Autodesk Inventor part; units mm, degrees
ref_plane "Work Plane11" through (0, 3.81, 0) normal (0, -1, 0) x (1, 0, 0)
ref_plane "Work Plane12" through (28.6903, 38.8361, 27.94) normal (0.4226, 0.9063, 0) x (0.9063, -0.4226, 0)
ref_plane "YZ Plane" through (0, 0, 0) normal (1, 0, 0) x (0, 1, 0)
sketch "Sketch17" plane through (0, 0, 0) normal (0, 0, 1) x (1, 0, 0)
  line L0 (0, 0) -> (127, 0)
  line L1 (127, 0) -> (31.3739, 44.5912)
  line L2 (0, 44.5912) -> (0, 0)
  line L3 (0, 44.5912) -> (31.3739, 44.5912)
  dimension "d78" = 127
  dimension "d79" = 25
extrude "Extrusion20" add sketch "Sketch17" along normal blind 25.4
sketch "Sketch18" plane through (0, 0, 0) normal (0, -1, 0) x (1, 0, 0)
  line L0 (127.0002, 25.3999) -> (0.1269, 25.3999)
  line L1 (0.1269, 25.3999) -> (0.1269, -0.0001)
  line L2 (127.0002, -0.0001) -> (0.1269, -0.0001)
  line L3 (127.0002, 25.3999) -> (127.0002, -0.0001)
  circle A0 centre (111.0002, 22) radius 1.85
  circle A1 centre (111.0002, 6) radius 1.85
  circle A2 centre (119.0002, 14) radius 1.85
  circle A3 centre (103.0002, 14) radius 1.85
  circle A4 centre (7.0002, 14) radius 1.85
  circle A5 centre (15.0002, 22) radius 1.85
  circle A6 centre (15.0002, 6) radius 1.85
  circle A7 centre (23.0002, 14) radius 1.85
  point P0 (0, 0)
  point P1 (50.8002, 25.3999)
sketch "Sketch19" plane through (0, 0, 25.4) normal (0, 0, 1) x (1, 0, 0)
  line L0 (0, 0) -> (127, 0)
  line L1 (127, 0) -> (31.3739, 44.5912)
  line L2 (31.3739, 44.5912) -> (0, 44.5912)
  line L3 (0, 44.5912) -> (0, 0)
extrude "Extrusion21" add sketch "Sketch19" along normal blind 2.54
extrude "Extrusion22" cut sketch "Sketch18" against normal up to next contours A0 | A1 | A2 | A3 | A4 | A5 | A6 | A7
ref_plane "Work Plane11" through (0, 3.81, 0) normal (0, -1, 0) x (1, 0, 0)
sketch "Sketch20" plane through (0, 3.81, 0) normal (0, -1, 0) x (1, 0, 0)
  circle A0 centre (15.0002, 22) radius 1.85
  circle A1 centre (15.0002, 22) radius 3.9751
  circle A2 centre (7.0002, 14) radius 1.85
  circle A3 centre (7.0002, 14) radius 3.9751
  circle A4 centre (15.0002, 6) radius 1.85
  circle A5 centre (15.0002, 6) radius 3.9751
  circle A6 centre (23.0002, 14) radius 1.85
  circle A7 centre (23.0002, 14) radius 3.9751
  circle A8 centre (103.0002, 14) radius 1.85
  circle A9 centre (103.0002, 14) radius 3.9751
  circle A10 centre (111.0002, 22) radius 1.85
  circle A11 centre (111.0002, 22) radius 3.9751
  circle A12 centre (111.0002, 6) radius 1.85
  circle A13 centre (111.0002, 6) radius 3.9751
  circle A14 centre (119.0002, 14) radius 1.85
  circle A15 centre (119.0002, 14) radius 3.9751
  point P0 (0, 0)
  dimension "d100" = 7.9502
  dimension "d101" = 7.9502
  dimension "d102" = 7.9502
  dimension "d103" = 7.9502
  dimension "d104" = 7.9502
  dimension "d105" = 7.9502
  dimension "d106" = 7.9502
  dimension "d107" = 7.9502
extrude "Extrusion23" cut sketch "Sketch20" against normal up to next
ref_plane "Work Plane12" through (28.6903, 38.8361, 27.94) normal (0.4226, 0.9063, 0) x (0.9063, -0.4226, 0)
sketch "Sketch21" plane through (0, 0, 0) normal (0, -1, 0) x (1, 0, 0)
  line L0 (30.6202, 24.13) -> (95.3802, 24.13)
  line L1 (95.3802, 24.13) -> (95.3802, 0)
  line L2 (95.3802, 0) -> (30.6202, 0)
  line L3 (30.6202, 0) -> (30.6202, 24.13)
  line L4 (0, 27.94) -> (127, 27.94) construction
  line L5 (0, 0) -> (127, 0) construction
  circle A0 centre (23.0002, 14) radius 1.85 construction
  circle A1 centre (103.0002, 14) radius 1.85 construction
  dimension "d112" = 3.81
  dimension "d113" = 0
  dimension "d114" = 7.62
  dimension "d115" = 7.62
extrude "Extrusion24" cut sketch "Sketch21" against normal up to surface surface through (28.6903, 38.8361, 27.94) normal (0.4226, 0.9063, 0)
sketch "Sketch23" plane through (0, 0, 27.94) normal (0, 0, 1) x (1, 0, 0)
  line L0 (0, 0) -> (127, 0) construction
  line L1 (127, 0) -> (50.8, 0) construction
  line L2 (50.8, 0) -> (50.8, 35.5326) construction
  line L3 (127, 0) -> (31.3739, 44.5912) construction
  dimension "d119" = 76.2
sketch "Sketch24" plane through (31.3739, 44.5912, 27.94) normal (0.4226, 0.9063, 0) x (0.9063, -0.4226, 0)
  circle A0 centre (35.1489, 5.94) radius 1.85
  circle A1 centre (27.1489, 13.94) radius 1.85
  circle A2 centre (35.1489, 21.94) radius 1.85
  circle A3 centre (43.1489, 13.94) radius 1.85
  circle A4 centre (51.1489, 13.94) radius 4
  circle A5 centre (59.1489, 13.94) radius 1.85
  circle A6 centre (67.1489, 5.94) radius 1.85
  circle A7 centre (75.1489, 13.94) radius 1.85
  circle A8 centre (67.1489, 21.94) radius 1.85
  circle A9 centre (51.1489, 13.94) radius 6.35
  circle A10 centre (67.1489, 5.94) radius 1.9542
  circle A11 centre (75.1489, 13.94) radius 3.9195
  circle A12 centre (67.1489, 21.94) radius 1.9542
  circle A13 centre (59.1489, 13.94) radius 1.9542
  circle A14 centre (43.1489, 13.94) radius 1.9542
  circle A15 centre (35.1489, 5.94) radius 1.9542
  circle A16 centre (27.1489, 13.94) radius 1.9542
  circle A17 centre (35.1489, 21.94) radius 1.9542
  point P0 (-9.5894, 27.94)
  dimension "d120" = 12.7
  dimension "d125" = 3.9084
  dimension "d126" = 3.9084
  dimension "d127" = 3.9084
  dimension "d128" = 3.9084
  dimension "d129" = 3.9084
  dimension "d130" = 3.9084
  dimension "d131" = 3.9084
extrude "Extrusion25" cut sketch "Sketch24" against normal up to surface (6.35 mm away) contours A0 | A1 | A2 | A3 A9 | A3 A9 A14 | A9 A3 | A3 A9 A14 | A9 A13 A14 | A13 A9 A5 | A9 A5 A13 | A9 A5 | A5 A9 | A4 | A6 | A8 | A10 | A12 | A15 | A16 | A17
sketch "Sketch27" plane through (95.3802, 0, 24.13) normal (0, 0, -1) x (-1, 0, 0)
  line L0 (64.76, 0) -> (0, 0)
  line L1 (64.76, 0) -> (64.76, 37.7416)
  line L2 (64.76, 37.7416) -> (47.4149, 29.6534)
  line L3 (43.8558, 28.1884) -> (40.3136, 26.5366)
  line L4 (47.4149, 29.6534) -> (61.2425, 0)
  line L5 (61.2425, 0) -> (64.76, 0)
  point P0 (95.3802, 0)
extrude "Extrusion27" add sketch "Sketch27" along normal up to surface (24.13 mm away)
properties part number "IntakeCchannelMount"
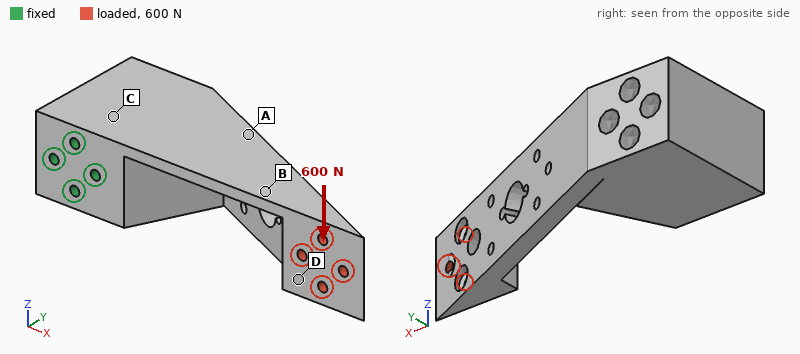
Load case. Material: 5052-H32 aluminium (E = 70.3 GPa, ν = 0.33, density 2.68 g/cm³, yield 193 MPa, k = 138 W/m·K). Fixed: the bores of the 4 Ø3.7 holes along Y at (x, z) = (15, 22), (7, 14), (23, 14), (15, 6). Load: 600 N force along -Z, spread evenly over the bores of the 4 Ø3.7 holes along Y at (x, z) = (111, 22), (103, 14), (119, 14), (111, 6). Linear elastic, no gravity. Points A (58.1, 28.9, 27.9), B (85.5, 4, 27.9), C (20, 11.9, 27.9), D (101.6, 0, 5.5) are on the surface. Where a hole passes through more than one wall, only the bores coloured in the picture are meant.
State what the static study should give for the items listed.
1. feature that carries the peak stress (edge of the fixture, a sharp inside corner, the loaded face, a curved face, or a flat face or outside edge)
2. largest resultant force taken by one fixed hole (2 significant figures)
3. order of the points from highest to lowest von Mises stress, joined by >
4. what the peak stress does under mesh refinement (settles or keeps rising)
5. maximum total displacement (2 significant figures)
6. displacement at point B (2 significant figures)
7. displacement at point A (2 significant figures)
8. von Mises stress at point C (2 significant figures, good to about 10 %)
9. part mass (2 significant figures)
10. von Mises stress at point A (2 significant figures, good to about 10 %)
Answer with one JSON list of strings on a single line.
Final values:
["edge of the fixture", "1.8 kN", "A > C > B > D", "keeps rising", "0.32 mm", "0.17 mm", "0.062 mm", "18 MPa", "170 g", "35 MPa"]
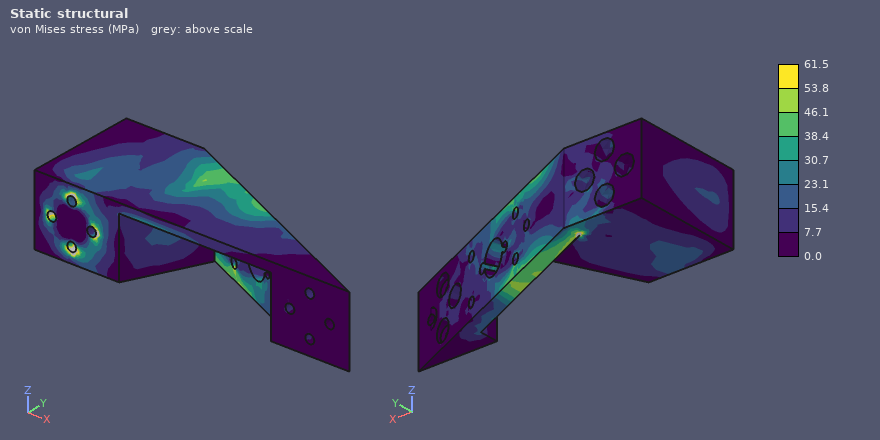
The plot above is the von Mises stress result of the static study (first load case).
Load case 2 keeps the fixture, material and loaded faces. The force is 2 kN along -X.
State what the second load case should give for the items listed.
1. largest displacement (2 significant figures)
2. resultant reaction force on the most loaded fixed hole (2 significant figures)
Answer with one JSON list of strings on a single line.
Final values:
["0.69 mm", "680 N"]
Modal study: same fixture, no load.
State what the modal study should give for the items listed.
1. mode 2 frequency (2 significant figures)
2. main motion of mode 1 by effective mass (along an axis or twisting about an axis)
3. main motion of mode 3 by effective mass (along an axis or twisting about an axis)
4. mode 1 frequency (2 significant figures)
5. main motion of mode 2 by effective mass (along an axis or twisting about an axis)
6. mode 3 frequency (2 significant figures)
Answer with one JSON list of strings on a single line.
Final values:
["1800 Hz", "along Y", "along X", "1400 Hz", "along Z", "2800 Hz"]
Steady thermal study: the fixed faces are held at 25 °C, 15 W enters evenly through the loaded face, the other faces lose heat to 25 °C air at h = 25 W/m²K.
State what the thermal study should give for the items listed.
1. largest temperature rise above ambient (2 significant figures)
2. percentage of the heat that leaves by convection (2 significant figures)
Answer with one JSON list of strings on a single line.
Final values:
["39 K", "36 %"]
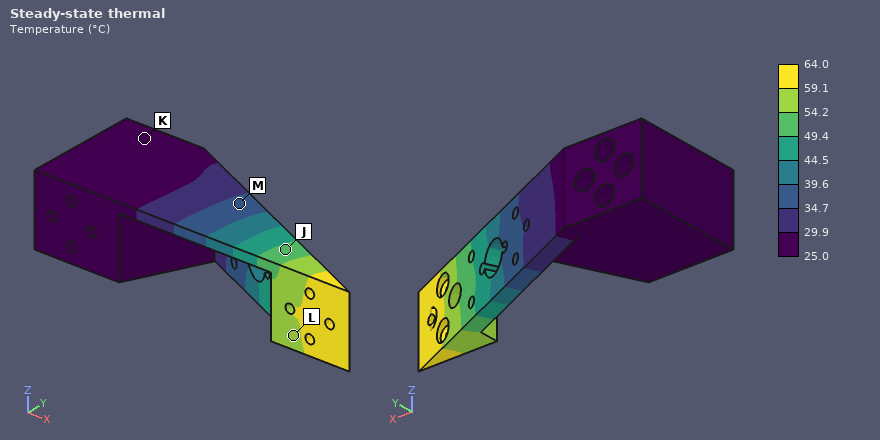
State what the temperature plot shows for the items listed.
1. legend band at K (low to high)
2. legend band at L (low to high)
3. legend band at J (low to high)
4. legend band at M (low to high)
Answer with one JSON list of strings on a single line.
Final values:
["25.0 to 29.9 °C", "54.2 to 59.1 °C", "49.4 to 54.2 °C", "34.7 to 39.6 °C"]
